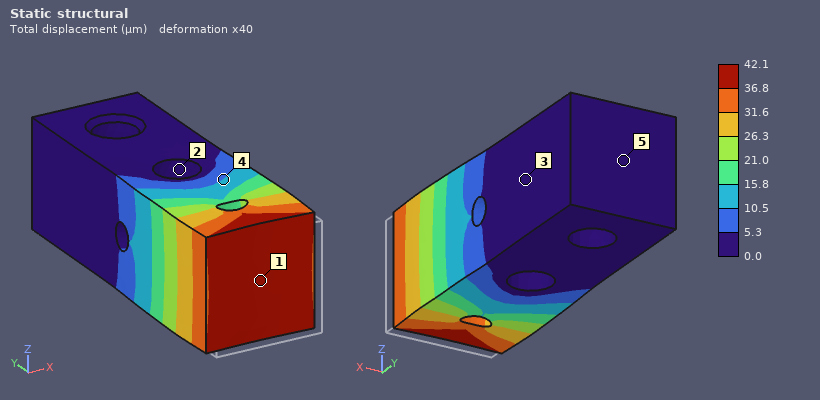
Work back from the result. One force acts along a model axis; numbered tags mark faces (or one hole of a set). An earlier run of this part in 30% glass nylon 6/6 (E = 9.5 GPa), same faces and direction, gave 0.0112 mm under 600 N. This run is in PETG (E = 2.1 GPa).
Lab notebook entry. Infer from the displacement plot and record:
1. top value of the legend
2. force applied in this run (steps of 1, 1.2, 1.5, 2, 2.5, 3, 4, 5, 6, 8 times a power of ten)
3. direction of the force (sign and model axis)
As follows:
42.1 µm
500 N
+Y
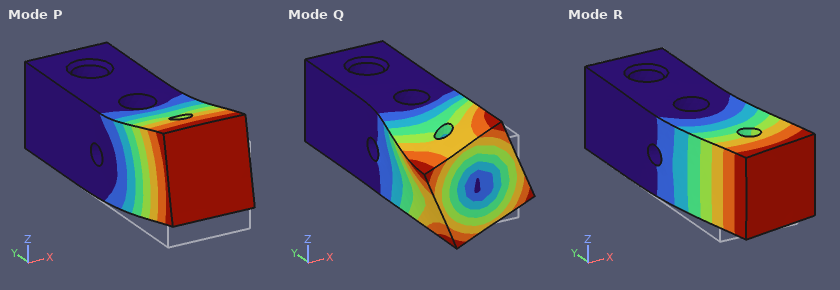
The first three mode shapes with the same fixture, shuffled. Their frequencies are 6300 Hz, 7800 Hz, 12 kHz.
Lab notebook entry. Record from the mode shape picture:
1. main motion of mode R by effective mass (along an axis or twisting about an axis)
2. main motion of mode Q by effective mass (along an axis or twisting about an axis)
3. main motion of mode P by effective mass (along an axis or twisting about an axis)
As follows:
along X
twisting about Y
along Z
